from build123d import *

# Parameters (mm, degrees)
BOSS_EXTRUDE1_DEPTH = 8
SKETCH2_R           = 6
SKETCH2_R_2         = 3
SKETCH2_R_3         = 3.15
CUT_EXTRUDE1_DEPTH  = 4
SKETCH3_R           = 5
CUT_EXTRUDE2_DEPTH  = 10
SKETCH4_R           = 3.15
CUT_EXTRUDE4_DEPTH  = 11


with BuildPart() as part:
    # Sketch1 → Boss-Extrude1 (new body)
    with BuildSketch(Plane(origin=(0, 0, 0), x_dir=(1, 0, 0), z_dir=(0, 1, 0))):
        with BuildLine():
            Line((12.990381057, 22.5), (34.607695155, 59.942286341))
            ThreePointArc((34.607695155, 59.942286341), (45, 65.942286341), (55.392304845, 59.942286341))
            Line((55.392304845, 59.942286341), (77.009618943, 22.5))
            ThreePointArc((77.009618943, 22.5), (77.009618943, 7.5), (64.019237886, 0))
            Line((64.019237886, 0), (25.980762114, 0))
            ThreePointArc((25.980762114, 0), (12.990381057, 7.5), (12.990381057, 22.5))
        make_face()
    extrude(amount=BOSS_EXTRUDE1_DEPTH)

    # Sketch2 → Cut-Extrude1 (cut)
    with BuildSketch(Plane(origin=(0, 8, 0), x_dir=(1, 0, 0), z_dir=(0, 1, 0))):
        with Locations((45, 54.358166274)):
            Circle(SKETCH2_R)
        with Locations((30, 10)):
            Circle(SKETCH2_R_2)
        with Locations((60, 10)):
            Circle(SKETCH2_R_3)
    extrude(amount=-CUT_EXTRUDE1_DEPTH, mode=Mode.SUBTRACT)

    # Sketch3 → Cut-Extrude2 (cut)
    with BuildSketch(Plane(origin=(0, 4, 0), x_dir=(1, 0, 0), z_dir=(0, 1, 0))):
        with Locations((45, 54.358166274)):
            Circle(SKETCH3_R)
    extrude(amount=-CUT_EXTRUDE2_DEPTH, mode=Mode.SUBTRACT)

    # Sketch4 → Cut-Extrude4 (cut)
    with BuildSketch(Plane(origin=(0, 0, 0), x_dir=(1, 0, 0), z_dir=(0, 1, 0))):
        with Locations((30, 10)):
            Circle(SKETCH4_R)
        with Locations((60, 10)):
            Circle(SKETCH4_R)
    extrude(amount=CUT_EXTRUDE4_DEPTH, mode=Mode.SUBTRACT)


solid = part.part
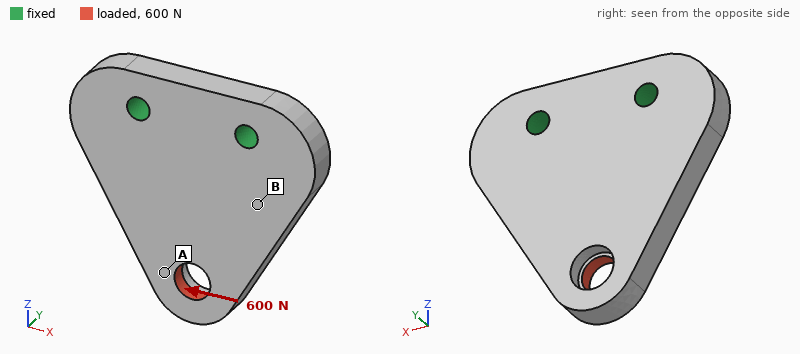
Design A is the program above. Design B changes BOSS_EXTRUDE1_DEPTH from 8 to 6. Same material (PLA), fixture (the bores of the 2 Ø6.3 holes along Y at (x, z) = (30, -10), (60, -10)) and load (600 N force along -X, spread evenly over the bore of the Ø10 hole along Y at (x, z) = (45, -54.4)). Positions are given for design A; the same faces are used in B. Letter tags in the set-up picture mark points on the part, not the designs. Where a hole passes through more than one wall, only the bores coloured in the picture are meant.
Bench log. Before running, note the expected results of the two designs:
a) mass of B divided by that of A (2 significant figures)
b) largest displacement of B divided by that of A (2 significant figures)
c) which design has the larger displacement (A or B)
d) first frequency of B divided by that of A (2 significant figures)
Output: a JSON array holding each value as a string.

["0.75", "1.3", "B", "0.77"]
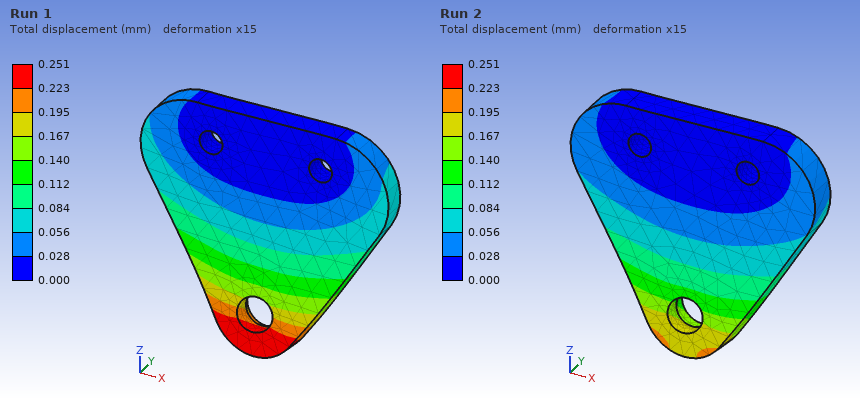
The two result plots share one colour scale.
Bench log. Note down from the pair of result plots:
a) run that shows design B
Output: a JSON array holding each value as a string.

["Run 1"]
